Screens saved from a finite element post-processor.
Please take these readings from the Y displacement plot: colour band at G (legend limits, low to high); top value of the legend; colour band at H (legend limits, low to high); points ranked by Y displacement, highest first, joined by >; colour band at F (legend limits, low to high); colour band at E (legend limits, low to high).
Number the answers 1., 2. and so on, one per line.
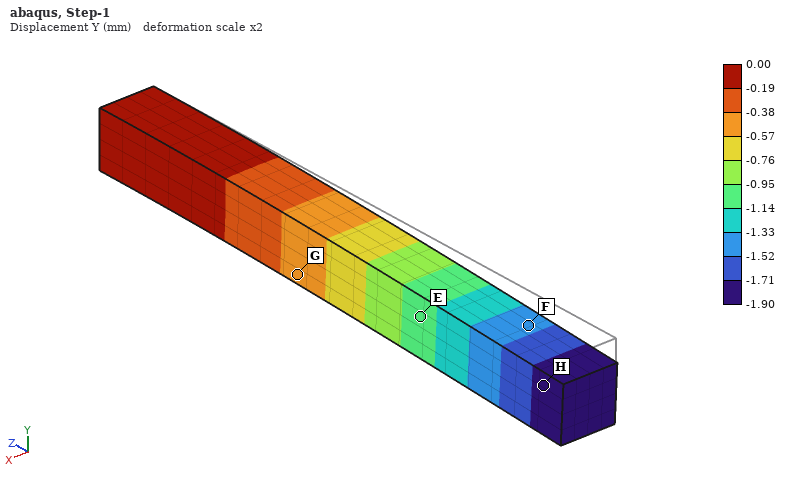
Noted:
1. -0.57 to -0.38 mm
2. 0.00 mm
3. -1.90 to -1.71 mm
4. G > E > F > H
5. -1.52 to -1.33 mm
6. -1.14 to -0.95 mm
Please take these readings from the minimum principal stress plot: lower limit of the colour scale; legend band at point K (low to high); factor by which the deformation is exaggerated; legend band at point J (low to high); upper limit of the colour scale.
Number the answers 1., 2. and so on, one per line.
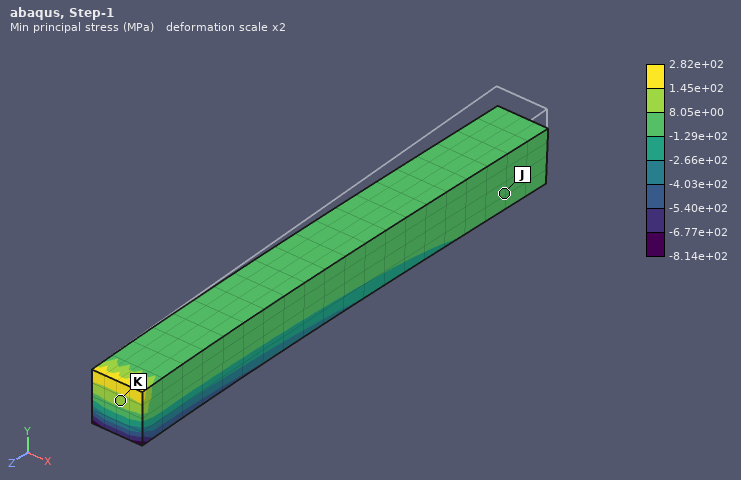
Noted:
1. -8.14e+02 MPa
2. 8.05e+00 to 1.45e+02 MPa
3. 2
4. -1.29e+02 to 8.05e+00 MPa
5. 2.82e+02 MPa
